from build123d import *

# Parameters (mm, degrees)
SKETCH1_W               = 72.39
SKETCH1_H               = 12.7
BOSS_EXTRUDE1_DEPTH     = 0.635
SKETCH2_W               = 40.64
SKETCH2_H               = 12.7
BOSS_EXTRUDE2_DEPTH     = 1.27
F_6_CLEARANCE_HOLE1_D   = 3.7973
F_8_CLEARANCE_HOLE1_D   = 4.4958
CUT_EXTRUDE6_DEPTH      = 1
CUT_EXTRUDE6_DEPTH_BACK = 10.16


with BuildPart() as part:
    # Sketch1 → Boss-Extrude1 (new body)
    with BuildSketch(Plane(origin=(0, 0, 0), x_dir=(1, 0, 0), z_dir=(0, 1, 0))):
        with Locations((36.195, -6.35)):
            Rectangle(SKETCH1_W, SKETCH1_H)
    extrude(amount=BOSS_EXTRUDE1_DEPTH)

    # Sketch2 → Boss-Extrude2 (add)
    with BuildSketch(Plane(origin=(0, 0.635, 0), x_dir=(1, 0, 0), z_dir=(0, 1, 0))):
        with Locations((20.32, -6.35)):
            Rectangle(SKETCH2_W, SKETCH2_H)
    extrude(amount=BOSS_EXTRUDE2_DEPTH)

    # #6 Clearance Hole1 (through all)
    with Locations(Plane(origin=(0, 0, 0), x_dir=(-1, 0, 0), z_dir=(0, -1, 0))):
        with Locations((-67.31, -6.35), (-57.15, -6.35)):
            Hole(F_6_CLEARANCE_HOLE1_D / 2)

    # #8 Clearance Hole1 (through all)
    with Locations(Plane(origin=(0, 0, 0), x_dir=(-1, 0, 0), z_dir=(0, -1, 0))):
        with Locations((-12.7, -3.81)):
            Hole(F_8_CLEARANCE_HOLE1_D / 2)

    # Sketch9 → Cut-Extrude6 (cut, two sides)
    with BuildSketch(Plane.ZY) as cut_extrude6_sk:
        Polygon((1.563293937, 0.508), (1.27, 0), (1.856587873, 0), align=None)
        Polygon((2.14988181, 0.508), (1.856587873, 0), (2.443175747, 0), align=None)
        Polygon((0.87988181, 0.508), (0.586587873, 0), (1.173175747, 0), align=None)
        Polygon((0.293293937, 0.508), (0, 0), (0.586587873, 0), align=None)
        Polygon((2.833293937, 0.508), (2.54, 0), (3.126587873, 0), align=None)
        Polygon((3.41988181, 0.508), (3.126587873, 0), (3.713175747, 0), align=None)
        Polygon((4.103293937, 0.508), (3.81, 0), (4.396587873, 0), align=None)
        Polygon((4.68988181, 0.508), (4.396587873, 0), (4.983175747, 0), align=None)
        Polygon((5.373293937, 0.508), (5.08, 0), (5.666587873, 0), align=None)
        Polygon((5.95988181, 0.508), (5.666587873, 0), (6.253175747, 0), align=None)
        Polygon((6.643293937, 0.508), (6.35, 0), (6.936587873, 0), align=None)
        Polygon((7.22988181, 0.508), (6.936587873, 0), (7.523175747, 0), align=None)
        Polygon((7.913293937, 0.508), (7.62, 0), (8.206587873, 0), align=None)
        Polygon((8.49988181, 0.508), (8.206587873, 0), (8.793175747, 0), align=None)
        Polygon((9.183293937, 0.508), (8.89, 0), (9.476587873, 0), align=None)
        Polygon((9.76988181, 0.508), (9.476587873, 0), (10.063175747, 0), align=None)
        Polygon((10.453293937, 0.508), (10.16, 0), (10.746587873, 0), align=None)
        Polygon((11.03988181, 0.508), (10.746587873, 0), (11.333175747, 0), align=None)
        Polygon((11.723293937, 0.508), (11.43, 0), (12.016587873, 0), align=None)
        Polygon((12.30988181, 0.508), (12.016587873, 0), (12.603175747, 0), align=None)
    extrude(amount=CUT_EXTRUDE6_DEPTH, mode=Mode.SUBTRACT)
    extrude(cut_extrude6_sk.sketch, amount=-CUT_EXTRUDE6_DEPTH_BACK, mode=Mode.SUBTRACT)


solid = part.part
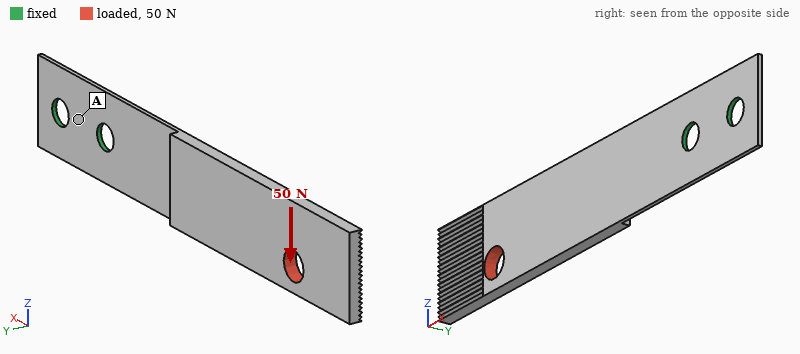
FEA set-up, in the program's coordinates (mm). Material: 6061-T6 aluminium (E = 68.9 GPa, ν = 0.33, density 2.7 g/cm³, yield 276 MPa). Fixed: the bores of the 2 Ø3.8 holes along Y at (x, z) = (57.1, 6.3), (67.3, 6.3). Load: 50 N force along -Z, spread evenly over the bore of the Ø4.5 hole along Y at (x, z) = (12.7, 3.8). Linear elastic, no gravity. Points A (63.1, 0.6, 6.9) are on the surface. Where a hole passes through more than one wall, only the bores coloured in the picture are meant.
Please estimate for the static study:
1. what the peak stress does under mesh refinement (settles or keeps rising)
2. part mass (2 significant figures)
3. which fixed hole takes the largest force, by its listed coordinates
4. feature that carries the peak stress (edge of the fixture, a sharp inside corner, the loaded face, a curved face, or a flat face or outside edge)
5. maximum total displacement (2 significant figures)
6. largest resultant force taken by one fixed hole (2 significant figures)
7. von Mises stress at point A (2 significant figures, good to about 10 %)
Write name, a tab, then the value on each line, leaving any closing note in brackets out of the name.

what the peak stress does under mesh refinement	keeps rising
part mass	3.1 g
which fixed hole takes the largest force, by its listed coordinates	(57.1, 6.3)
feature that carries the peak stress	edge of the fixture
maximum total displacement	0.33 mm
largest resultant force taken by one fixed hole	160 N
von Mises stress at point A	23 MPa
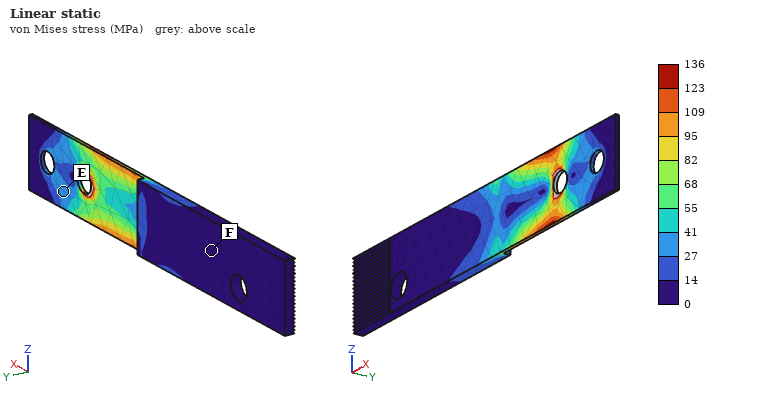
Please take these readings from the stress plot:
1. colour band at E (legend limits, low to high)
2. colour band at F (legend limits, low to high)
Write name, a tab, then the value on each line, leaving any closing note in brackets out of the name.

colour band at E	27 to 41 MPa
colour band at F	0 to 14 MPa
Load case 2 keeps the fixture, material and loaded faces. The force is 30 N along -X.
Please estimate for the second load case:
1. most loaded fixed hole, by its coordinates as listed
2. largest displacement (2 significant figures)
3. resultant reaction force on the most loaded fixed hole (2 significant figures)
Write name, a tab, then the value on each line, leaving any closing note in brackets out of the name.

most loaded fixed hole, by its coordinates as listed	(57.1, 6.3)
largest displacement	0.72 mm
resultant reaction force on the most loaded fixed hole	26 N
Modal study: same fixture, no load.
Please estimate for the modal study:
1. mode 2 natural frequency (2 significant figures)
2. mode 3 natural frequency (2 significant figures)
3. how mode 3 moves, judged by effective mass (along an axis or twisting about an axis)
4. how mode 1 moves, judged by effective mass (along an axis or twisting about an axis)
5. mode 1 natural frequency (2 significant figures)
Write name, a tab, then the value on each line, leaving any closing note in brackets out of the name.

mode 2 natural frequency	1200 Hz
mode 3 natural frequency	1600 Hz
how mode 3 moves, judged by effective mass	along Y
how mode 1 moves, judged by effective mass	along Y
mode 1 natural frequency	120 Hz
